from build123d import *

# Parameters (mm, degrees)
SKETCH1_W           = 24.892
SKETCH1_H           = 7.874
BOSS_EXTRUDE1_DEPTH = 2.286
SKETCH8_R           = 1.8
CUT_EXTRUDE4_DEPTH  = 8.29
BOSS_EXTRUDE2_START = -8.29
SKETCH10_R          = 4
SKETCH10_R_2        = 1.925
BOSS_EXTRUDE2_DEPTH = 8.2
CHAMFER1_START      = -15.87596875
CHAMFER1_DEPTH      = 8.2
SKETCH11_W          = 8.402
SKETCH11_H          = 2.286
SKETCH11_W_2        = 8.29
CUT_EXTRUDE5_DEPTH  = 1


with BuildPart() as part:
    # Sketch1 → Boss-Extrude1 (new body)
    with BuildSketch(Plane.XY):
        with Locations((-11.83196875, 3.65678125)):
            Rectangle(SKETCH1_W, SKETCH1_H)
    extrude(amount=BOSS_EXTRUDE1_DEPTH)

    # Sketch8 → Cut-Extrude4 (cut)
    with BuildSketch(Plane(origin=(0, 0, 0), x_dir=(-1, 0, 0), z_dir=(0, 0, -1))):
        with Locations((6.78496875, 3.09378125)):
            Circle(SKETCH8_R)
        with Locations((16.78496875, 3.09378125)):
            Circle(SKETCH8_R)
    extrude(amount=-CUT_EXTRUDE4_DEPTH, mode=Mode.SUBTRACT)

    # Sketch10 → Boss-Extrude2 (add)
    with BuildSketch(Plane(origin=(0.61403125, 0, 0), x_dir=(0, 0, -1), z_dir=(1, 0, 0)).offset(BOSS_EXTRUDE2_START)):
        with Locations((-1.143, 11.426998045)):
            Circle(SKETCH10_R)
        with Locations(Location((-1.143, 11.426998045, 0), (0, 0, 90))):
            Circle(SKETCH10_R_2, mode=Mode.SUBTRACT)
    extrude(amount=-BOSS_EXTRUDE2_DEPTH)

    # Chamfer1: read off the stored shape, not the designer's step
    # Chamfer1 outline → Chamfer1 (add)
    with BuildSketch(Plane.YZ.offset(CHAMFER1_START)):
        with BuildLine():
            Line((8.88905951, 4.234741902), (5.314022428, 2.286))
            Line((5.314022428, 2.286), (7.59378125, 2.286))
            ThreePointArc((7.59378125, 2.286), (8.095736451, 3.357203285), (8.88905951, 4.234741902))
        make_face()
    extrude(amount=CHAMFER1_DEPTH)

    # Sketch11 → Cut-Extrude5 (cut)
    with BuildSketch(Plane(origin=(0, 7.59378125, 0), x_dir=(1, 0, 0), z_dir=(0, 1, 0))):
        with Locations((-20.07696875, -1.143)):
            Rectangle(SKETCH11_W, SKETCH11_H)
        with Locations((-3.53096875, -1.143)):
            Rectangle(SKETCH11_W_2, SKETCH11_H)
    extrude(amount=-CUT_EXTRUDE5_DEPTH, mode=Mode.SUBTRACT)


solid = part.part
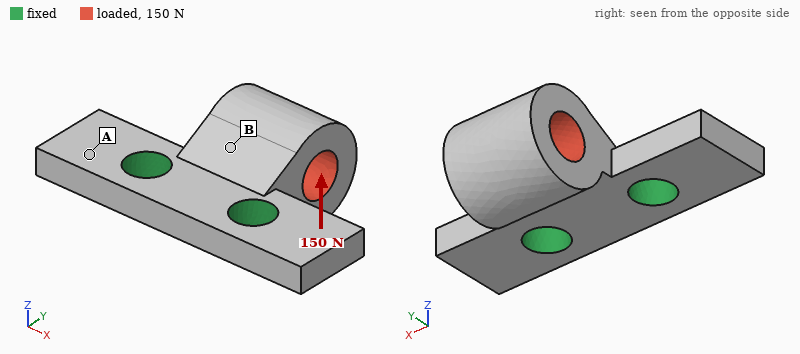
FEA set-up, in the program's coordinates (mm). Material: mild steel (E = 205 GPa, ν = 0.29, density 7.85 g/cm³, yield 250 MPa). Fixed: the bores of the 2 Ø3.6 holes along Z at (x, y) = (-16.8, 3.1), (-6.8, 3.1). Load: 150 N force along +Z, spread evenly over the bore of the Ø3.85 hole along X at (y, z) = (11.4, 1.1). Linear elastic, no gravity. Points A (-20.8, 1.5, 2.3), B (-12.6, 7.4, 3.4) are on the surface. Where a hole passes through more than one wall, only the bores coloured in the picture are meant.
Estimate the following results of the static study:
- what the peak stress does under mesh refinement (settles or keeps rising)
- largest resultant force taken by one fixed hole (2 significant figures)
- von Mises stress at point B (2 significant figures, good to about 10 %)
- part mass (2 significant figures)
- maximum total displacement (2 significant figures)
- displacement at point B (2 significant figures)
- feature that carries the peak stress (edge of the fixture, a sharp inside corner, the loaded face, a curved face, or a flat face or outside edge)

keeps rising
76 N
33 MPa
5.4 g
15 µm
4.3 µm
edge of the fixture
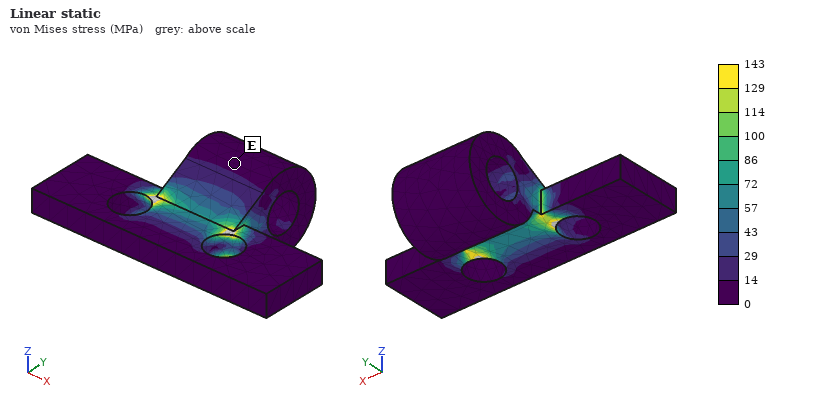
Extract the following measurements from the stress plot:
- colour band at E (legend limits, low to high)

0 to 14 MPa
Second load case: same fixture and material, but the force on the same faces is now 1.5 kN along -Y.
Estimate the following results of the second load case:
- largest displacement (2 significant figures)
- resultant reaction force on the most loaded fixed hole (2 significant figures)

6.0 µm
790 N
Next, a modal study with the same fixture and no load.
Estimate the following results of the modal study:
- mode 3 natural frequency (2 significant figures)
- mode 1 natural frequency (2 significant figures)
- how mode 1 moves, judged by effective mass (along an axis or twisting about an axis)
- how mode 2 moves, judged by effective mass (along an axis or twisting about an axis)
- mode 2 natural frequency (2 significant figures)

45 kHz
11 kHz
along Z
along X
34 kHz
